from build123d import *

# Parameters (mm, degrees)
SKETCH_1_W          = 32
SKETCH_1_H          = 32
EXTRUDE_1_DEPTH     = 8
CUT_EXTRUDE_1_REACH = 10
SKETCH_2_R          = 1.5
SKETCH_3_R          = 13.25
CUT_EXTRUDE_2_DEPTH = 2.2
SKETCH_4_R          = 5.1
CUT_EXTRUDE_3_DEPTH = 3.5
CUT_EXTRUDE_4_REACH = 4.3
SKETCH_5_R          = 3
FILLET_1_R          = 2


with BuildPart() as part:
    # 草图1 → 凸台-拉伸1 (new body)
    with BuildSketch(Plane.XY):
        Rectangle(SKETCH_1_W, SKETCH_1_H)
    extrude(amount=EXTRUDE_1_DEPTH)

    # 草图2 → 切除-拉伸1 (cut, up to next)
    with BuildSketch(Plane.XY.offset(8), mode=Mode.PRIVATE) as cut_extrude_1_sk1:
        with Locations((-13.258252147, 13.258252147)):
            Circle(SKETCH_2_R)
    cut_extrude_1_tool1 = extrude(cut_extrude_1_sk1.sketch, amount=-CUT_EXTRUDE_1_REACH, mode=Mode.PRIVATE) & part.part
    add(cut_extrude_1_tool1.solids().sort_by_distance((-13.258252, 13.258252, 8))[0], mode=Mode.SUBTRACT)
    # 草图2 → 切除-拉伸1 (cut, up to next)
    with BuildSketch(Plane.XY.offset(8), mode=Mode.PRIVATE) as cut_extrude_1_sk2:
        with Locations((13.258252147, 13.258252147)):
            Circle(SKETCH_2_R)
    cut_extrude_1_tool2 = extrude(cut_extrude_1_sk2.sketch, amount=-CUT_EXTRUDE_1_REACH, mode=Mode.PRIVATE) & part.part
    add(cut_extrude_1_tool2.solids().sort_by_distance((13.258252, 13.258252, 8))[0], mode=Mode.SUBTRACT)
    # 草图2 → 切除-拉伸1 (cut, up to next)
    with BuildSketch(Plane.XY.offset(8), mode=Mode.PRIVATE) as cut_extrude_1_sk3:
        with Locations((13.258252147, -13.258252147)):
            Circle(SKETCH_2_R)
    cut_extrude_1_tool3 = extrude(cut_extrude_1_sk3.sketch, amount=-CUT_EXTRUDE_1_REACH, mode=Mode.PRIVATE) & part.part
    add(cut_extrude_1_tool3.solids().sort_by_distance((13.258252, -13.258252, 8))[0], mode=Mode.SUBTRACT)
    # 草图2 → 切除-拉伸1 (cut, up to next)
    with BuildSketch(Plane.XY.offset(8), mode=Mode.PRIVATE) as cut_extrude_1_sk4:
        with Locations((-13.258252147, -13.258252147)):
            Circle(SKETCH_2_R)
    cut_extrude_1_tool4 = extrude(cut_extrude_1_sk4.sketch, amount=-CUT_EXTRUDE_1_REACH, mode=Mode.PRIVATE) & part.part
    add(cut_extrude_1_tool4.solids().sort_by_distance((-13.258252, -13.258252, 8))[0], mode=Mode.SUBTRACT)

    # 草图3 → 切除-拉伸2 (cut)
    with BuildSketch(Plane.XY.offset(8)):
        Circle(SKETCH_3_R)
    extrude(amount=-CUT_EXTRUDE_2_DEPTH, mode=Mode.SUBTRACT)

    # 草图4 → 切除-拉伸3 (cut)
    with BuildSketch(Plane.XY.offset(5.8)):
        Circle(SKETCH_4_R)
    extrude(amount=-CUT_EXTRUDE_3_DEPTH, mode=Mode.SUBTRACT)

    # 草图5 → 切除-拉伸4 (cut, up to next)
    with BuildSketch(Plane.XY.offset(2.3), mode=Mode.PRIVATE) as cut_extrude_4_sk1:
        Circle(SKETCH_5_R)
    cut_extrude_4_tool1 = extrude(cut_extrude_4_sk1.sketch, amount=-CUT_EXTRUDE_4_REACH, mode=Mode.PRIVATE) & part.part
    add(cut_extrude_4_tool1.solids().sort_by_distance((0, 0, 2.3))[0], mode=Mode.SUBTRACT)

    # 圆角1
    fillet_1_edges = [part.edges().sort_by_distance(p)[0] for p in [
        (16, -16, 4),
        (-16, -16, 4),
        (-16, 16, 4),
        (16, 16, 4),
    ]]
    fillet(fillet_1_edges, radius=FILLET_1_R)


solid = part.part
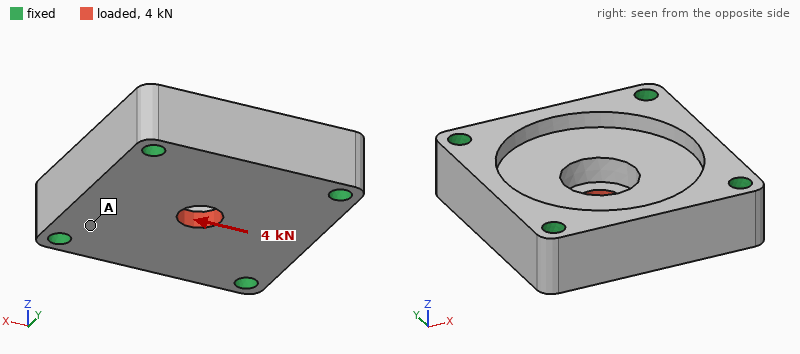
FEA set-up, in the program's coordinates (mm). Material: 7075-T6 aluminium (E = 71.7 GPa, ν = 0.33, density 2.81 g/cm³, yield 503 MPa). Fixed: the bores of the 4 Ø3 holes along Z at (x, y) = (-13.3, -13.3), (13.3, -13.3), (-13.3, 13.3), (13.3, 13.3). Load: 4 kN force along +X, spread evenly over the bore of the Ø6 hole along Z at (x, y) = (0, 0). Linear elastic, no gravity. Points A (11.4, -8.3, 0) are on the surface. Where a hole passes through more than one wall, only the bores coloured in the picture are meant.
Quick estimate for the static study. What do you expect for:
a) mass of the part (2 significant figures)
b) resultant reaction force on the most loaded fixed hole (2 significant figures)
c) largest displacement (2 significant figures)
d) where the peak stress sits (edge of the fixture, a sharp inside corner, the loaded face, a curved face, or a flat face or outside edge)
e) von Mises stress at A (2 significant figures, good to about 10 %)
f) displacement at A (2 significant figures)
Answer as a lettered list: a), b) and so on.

a) 18 g
b) 1.2 kN
c) 12 µm
d) a sharp inside corner
e) 27 MPa
f) 2.6 µm
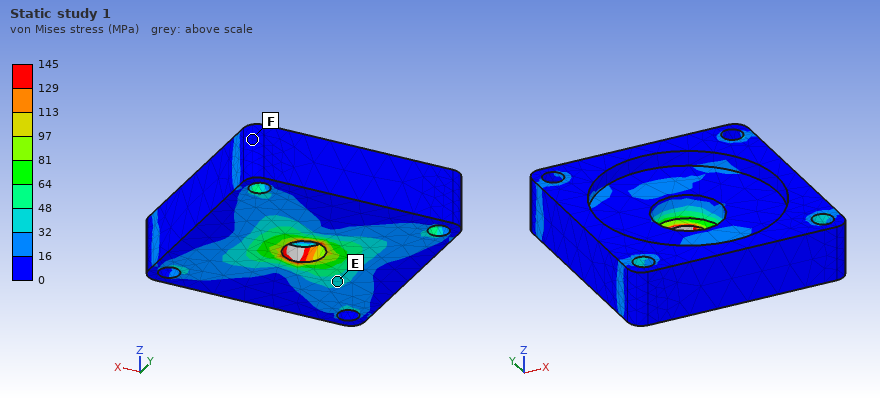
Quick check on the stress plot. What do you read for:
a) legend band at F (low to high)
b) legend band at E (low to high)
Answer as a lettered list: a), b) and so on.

a) 0 to 16 MPa
b) 32 to 48 MPa
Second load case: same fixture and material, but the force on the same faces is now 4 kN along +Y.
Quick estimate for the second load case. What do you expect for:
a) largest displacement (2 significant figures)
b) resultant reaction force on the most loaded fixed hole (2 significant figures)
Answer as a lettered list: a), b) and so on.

a) 12 µm
b) 1.2 kN
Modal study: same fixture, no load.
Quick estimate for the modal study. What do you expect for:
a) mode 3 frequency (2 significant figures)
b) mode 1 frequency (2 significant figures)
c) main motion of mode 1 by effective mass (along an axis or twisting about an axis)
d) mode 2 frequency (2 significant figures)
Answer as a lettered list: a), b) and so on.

a) 42 kHz
b) 30 kHz
c) along Z
d) 42 kHz
